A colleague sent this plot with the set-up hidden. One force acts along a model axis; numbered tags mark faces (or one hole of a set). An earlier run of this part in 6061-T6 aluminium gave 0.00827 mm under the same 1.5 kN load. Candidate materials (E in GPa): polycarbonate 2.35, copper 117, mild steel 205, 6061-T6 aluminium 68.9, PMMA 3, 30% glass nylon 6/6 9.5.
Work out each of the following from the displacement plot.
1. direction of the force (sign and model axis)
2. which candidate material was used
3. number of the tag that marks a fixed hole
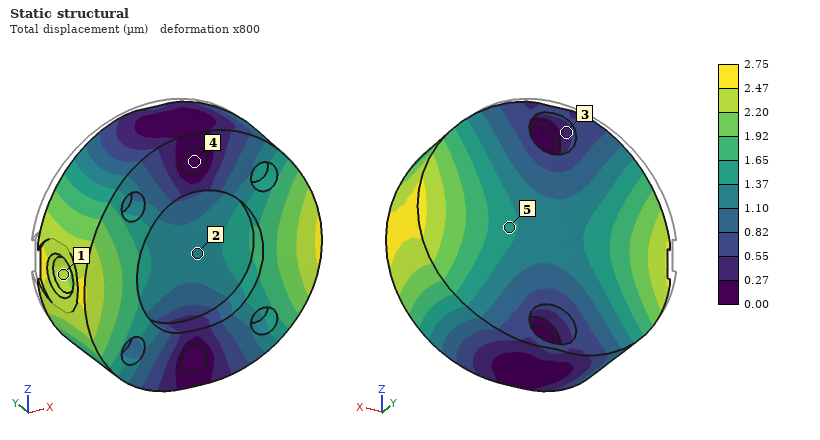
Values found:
-Y
mild steel
4
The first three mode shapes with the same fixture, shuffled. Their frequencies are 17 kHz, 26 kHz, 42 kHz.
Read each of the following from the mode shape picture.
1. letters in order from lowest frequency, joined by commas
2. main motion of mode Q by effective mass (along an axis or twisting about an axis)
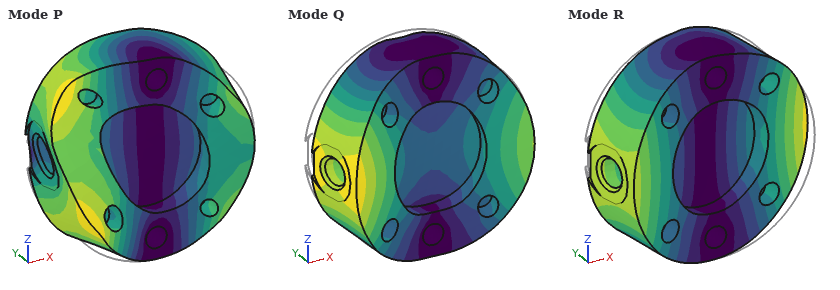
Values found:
R, Q, P
along Y
